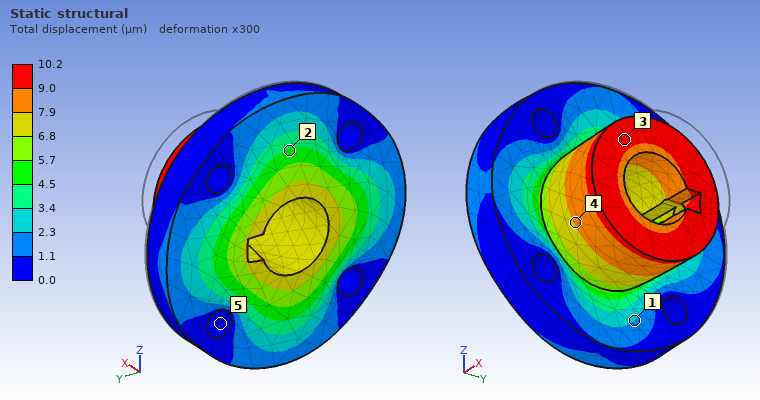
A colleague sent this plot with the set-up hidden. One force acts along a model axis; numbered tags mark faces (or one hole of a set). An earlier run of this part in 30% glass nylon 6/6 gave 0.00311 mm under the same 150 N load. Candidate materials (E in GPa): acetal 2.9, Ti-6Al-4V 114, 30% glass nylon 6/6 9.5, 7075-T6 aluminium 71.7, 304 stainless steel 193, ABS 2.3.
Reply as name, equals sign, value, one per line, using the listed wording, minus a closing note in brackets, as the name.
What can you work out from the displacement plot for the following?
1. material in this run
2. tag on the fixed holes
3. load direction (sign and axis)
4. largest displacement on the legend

material in this run = acetal
tag on the fixed holes = 5
load direction = -X
largest displacement on the legend = 10.2 µm
